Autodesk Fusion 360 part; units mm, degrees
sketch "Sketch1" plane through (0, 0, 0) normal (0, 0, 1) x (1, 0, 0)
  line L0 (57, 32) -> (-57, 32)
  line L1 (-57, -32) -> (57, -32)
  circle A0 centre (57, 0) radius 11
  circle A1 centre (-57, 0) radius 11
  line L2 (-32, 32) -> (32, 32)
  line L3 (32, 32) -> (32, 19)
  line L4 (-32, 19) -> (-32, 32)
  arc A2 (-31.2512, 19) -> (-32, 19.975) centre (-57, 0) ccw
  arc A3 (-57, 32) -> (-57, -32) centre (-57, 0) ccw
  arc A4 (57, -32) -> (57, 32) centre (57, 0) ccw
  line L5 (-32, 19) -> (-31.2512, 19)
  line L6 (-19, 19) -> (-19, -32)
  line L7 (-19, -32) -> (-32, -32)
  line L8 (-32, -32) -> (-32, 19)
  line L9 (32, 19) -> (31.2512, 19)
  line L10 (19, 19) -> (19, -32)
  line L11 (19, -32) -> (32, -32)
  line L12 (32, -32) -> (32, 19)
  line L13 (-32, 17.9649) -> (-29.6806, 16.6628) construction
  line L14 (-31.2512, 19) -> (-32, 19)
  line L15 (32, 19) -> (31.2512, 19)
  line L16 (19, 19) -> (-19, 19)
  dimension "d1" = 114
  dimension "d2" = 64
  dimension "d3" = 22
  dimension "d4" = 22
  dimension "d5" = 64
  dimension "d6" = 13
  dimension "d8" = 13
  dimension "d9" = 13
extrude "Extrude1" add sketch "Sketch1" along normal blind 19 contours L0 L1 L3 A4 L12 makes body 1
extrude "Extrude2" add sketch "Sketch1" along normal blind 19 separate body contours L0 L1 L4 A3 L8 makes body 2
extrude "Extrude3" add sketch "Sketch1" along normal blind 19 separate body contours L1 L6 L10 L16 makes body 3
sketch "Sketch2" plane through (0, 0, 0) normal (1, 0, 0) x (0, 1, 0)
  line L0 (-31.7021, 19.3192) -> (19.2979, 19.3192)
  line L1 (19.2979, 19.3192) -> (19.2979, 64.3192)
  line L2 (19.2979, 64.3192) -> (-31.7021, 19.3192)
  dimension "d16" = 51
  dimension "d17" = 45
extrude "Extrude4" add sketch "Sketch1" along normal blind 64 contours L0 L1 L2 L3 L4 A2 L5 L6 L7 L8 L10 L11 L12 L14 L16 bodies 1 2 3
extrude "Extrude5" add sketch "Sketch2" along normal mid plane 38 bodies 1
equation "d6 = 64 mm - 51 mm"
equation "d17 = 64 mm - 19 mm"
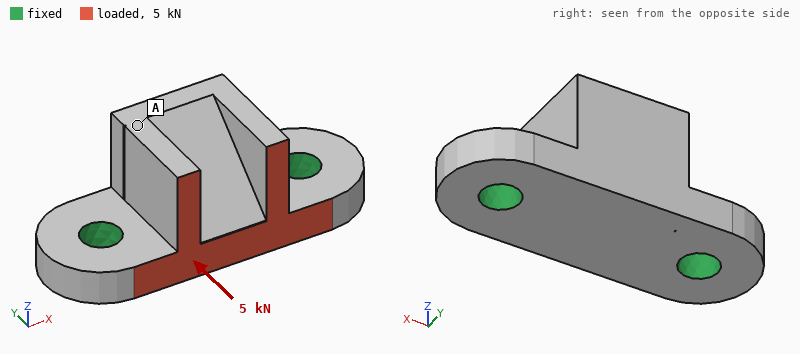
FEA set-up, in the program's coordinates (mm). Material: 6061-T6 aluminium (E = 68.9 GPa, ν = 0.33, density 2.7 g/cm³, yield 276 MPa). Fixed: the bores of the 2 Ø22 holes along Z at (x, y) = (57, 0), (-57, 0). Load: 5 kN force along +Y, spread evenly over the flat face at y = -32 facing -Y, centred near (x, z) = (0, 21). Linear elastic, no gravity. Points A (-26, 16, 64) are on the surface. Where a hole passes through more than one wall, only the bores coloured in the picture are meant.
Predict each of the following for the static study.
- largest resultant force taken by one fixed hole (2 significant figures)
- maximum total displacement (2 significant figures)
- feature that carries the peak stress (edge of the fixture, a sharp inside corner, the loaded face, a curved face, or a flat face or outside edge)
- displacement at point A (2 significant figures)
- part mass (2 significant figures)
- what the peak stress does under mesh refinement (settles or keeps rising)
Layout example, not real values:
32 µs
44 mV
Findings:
2.5 kN
15 µm
edge of the fixture
13 µm
880 g
keeps rising
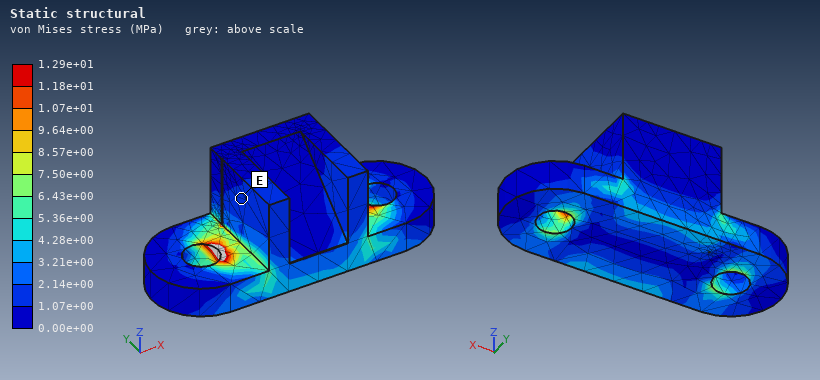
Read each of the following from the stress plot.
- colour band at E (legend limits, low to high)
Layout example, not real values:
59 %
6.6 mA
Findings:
1.07e+00 to 2.14e+00 MPa
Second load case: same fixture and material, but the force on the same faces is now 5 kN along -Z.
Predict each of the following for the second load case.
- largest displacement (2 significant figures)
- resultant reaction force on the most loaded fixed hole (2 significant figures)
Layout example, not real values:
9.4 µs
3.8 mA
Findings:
30 µm
2.6 kN
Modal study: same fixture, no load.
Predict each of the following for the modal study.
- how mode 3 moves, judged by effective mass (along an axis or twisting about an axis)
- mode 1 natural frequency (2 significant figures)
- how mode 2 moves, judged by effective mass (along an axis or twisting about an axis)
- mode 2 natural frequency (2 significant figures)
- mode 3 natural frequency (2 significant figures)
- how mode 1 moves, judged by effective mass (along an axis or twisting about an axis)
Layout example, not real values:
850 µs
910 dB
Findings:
along X
3500 Hz
along Z
6300 Hz
7000 Hz
along Y
